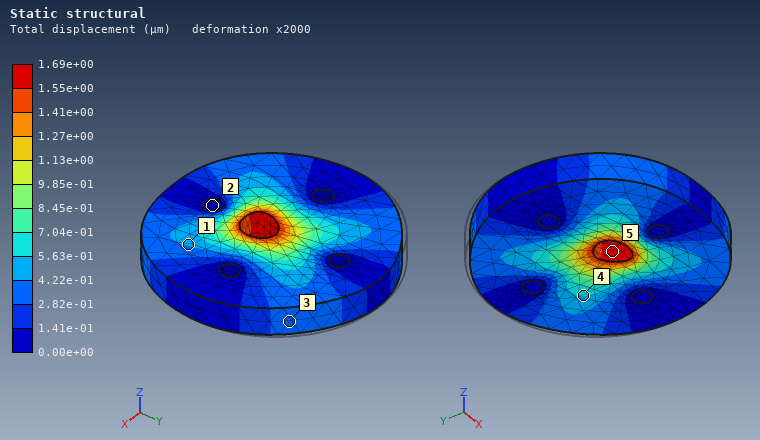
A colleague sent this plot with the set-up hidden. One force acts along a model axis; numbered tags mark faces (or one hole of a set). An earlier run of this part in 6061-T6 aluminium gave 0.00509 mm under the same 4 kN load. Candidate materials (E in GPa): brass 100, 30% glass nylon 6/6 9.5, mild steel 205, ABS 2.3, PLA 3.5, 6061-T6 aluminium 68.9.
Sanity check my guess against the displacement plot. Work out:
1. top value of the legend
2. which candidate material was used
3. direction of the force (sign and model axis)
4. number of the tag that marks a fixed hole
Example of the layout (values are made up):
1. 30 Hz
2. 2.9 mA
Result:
1. 1.69e+00 µm
2. mild steel
3. -Y
4. 2
